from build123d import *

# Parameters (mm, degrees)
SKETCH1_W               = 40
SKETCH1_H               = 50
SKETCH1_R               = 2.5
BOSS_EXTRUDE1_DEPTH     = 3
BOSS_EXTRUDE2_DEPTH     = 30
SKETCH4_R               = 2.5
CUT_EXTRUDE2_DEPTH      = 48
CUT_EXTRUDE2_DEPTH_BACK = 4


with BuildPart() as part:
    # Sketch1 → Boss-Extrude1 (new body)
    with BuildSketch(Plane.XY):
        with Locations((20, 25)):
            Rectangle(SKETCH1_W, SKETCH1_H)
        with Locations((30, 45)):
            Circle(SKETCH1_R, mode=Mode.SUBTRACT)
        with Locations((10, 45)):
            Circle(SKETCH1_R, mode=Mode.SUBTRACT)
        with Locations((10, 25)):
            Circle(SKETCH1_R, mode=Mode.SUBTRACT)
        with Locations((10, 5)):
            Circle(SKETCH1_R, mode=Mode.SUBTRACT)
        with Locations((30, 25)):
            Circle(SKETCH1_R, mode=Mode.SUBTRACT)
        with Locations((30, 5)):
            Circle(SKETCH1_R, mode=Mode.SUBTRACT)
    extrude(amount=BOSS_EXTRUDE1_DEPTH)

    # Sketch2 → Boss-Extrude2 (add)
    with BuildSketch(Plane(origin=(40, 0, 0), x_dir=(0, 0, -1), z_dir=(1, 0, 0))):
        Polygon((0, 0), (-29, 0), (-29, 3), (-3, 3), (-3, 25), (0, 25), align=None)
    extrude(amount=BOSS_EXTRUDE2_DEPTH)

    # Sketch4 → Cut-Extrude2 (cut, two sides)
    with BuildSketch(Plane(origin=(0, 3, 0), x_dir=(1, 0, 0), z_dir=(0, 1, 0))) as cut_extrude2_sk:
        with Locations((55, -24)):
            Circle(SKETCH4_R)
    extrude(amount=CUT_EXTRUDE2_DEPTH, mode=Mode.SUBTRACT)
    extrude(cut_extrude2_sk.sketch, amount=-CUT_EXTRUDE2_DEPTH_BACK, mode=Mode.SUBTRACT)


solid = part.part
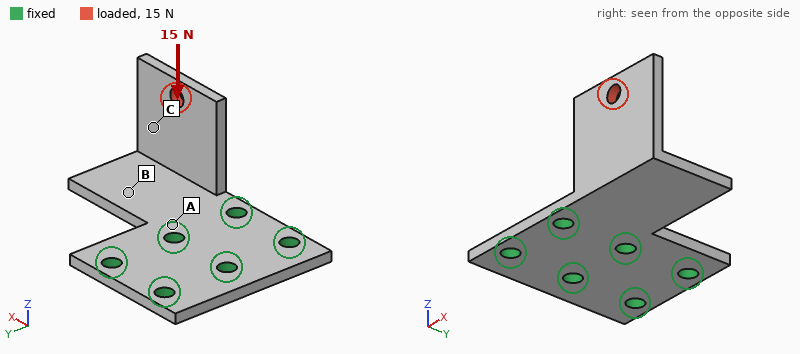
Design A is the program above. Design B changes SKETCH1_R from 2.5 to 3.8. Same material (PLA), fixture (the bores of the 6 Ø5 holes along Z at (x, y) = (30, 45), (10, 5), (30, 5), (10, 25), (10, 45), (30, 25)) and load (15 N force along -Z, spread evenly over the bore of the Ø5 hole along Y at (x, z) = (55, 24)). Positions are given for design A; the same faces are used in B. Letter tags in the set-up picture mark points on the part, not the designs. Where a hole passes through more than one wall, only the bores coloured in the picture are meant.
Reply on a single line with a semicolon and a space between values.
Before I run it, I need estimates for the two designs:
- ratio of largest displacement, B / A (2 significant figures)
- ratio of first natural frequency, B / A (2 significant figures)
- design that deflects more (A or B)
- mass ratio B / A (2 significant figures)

0.86; 1.1; A; 0.95
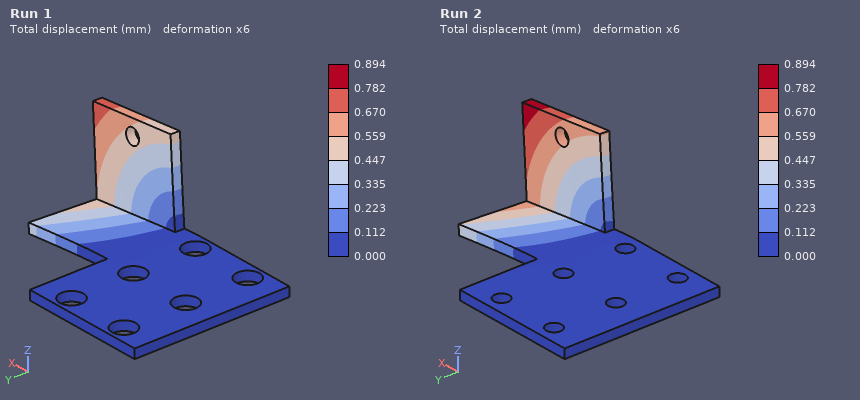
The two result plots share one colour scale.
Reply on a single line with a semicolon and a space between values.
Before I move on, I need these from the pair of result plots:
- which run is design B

Run 1
